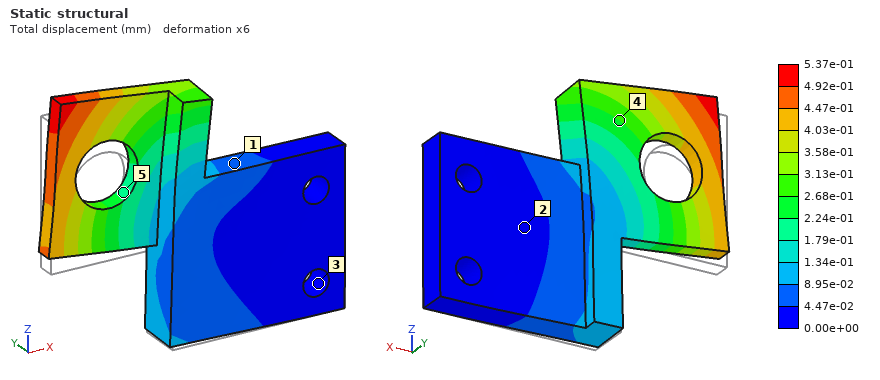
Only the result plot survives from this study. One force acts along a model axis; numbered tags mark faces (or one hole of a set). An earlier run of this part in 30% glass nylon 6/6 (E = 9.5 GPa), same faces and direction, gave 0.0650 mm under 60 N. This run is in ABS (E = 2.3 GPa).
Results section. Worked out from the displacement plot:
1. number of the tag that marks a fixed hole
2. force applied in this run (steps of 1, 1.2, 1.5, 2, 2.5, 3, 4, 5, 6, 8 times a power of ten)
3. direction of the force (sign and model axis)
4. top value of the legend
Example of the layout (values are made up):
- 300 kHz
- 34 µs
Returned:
- 3
- 120 N
- +Z
- 5.37e-01 mm
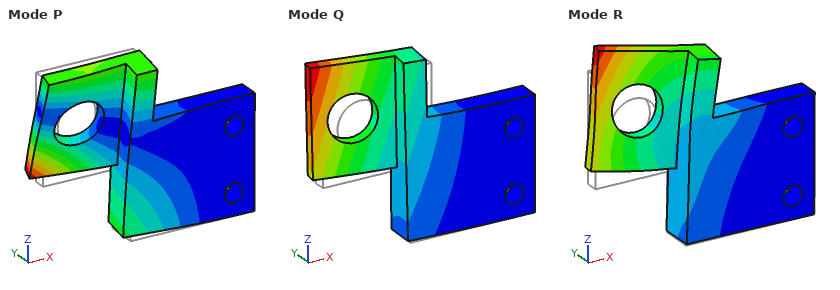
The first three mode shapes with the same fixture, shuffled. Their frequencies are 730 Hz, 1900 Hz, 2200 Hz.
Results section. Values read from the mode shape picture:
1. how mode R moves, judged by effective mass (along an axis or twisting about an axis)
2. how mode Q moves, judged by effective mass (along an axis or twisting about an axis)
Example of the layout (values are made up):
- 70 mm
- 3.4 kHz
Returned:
- along Z
- along Y
